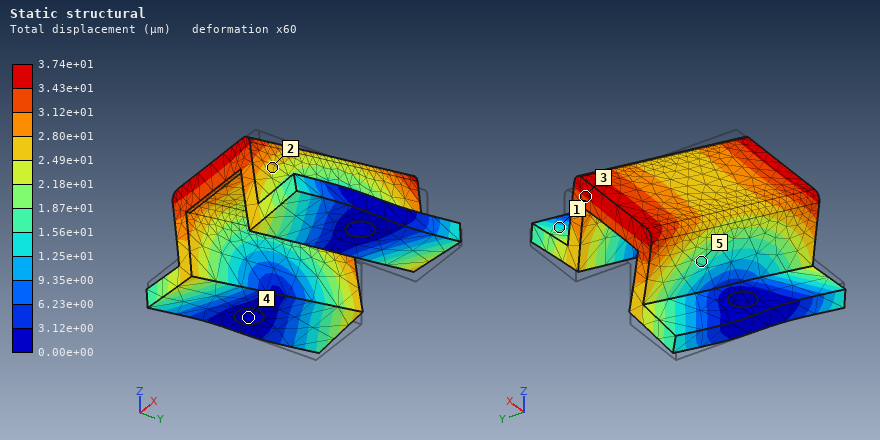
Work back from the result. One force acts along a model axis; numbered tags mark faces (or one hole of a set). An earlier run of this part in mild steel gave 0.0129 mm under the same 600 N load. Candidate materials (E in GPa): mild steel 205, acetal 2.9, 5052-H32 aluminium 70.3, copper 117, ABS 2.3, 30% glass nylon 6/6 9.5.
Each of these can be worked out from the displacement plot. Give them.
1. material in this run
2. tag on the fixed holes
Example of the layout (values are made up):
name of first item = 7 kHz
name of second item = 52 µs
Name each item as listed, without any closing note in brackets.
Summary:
material in this run = 5052-H32 aluminium
tag on the fixed holes = 4
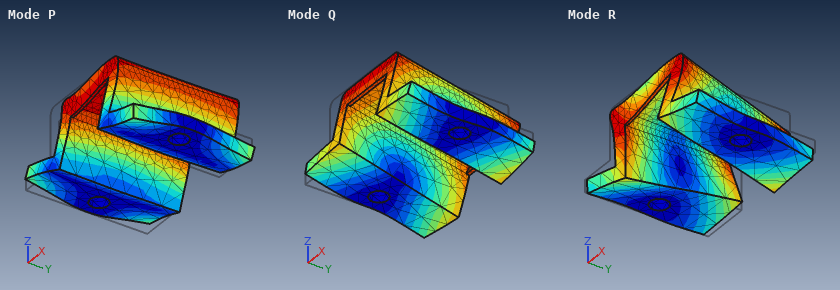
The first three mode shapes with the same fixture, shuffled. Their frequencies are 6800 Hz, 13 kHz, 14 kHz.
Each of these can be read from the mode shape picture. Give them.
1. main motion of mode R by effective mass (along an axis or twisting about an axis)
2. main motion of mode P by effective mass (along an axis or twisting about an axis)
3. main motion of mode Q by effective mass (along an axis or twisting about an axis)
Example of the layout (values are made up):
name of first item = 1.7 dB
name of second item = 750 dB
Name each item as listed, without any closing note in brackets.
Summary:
main motion of mode R by effective mass = twisting about Z
main motion of mode P by effective mass = along X
main motion of mode Q by effective mass = along Y
